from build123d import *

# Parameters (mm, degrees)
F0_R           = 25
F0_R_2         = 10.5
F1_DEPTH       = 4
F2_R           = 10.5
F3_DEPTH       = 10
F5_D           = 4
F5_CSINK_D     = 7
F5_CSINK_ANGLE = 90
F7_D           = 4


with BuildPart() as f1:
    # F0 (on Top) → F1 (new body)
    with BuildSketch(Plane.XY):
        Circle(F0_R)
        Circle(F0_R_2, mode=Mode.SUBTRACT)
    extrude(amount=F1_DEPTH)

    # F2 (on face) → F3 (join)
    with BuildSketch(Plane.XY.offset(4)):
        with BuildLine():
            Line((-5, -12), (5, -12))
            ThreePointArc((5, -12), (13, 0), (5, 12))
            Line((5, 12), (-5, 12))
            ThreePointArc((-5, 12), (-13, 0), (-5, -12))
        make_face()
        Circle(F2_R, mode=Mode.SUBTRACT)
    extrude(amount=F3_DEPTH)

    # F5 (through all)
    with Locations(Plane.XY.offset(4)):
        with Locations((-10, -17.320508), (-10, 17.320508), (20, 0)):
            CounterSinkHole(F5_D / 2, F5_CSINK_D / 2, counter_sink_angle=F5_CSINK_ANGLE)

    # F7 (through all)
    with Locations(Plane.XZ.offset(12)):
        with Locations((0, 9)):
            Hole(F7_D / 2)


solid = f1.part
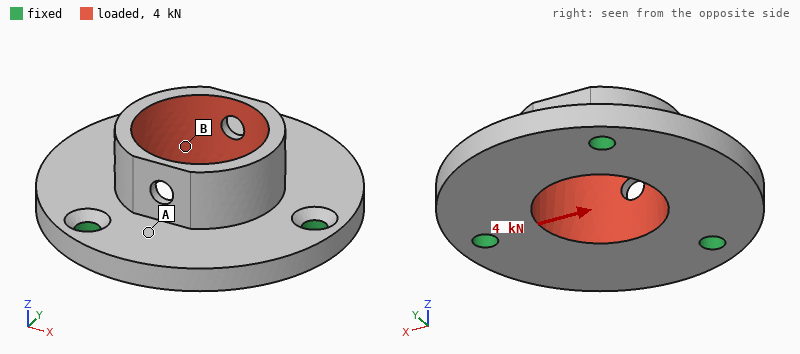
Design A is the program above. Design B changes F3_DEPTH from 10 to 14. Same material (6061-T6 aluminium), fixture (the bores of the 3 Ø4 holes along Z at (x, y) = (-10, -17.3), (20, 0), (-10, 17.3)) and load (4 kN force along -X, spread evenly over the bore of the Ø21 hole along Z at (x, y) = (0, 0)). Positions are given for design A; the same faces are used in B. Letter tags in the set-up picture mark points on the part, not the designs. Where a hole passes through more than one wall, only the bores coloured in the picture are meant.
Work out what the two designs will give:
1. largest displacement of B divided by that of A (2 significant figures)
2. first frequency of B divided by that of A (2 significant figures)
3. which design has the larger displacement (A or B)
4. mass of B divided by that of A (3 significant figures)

1.4
0.98
B
1.09
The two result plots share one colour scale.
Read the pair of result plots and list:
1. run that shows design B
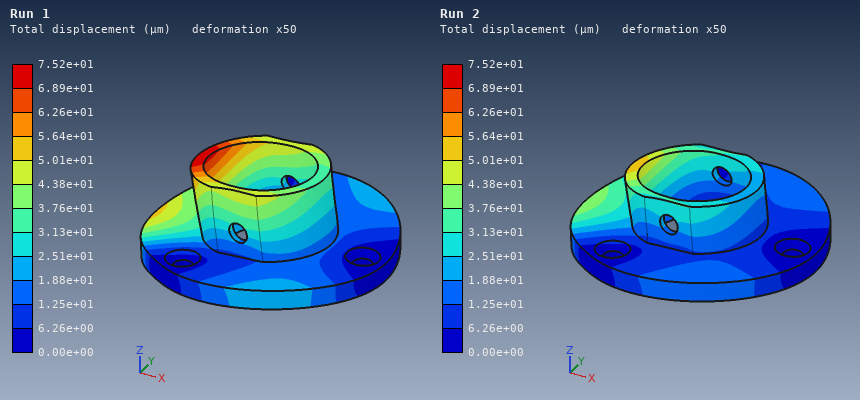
Run 1
